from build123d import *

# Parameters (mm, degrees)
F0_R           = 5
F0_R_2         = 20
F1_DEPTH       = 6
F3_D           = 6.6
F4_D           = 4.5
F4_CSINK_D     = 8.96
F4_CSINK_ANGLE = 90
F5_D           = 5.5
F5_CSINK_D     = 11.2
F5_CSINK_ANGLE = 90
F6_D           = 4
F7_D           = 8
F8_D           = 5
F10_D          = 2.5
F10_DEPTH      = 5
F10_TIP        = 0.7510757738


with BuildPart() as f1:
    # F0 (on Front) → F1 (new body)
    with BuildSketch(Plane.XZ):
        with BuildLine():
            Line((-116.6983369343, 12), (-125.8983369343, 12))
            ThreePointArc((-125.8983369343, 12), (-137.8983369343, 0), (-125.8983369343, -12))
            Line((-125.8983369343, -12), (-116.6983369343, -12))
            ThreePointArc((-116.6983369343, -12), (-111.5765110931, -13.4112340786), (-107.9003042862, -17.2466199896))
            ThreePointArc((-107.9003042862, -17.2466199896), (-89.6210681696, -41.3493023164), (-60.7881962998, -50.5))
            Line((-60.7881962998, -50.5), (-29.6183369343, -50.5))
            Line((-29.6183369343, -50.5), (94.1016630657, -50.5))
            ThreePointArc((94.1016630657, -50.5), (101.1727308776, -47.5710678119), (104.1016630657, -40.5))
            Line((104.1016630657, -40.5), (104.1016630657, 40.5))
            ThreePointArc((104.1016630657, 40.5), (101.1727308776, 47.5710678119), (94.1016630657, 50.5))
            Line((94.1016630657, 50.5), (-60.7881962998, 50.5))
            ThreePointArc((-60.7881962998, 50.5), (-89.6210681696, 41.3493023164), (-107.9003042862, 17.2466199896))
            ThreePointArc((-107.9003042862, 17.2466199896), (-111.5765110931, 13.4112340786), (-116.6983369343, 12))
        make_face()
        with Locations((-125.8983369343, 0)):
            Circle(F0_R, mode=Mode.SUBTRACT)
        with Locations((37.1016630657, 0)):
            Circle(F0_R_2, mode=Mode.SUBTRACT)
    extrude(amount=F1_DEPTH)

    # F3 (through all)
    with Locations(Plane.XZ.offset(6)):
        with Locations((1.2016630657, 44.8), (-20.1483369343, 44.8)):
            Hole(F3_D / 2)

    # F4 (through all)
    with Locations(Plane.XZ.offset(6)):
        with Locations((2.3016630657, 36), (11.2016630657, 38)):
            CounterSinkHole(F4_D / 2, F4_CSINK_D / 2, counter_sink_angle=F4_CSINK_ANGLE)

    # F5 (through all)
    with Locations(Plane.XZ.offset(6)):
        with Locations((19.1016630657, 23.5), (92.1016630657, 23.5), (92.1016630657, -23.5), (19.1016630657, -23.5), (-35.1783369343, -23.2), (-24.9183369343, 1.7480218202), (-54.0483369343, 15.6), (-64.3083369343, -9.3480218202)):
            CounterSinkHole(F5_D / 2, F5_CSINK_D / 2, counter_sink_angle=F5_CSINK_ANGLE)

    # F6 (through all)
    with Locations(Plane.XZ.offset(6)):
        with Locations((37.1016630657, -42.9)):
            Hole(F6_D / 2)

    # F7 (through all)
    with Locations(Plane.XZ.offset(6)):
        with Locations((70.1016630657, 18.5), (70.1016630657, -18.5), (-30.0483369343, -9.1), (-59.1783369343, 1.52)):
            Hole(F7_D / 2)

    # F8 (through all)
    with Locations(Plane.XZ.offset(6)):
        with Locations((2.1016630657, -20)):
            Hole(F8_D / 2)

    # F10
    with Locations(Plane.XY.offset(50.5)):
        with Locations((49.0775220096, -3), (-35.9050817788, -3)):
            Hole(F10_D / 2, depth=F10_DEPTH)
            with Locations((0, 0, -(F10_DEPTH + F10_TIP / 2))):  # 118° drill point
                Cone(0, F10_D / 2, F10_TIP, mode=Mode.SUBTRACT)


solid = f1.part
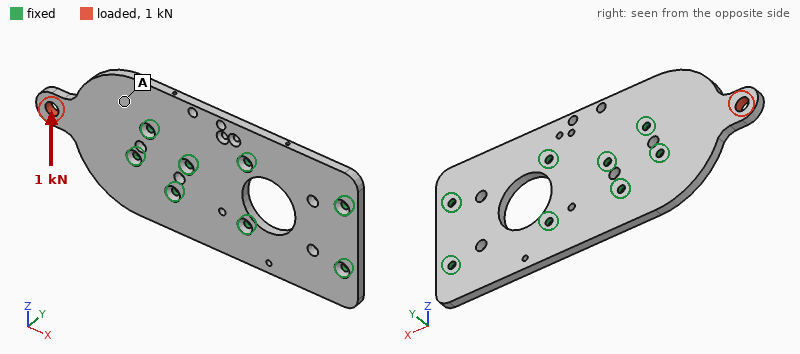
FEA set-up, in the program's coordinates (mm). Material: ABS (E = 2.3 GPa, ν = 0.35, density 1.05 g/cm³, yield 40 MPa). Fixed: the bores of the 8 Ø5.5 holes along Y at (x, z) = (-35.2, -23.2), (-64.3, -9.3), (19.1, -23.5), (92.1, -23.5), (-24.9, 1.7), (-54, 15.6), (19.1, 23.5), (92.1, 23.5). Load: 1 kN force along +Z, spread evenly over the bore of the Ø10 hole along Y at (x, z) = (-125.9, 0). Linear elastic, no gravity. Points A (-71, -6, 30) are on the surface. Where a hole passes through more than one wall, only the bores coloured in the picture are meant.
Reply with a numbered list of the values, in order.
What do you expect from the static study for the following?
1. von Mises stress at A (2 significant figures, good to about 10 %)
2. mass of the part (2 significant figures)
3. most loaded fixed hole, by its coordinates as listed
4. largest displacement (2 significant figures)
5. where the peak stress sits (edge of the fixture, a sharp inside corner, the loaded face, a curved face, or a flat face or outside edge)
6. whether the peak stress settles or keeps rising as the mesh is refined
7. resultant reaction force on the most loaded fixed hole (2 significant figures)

1. 4.4 MPa
2. 120 g
3. (-64.3, -9.3)
4. 1.1 mm
5. edge of the fixture
6. keeps rising
7. 980 N
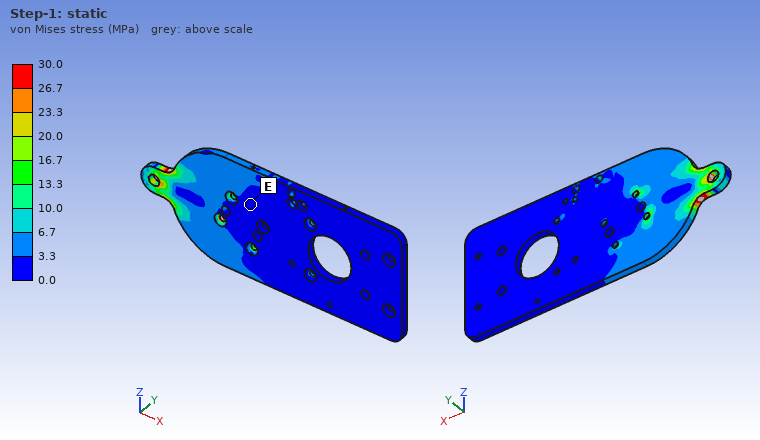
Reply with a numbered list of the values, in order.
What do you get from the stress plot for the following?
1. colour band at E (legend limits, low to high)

1. 0.0 to 3.3 MPa
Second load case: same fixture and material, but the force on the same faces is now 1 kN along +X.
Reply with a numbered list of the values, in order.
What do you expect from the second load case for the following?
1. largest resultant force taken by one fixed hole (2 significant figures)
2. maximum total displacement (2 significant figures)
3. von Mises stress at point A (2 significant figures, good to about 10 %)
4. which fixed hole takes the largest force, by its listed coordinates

1. 390 N
2. 0.23 mm
3. 1.3 MPa
4. (-64.3, -9.3)
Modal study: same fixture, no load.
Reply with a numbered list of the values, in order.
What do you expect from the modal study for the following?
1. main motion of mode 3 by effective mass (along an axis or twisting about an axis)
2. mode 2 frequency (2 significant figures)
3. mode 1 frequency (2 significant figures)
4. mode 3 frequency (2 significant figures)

1. along Y
2. 790 Hz
3. 390 Hz
4. 980 Hz
